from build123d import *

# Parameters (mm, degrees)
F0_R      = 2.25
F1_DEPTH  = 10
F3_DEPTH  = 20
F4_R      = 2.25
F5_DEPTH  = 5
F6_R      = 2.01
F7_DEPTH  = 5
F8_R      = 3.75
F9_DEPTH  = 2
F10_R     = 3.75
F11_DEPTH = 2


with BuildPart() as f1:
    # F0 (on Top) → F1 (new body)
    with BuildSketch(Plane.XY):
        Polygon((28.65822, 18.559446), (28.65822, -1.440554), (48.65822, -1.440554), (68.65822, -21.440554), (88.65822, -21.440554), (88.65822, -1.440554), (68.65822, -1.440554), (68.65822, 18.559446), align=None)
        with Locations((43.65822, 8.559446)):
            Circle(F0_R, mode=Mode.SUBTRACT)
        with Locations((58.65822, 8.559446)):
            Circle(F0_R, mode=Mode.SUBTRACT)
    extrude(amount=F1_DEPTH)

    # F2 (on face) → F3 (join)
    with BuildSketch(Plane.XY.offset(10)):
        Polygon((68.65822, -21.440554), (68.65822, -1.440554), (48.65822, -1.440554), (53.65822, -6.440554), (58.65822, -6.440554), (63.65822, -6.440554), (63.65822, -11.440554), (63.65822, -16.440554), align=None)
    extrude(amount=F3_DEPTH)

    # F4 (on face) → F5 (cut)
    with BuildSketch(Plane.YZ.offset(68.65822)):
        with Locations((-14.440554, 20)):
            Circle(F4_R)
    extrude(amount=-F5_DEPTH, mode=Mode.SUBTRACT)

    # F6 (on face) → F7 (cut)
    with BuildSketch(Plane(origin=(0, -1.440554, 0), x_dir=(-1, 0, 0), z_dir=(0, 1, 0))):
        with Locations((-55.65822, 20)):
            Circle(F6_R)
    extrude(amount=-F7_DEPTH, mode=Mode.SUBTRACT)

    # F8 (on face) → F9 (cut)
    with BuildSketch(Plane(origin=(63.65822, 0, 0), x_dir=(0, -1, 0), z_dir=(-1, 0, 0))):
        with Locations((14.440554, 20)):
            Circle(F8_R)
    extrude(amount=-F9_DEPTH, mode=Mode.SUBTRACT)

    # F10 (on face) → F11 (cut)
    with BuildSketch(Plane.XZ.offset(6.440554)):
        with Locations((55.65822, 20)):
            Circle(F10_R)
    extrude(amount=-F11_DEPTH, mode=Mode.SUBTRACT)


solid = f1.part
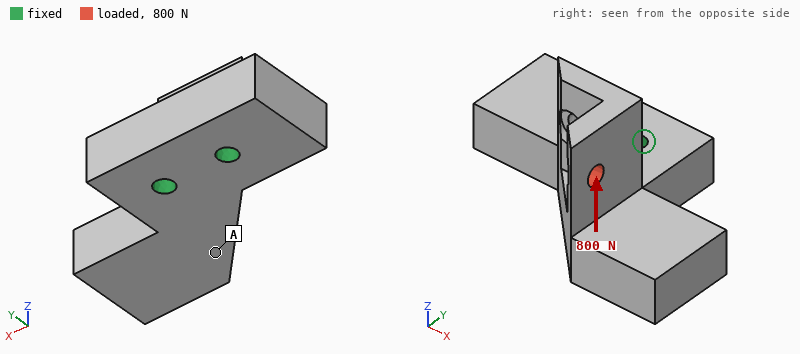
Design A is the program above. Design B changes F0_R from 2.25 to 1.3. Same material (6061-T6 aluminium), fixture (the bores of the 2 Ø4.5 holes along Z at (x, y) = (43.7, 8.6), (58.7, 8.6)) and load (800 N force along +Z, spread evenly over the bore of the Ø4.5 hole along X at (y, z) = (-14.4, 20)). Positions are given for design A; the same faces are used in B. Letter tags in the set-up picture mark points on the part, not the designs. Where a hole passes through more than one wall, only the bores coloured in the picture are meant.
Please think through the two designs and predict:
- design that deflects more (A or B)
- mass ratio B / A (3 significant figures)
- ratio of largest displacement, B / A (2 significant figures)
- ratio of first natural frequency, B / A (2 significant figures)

B
1.01
1.2
0.93
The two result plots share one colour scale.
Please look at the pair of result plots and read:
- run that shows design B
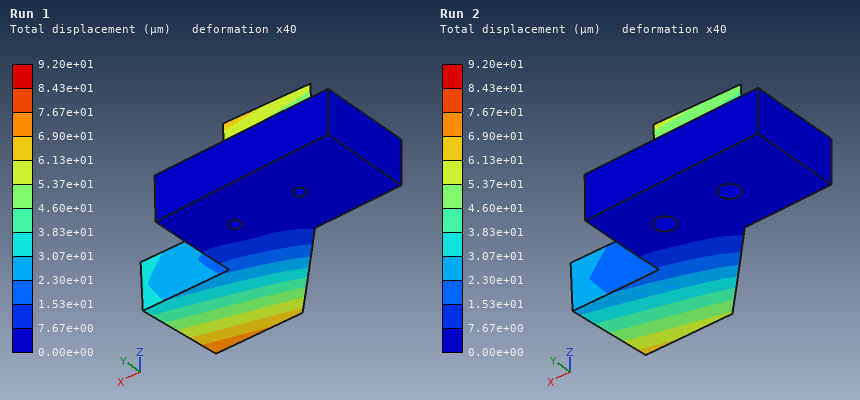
Run 1
